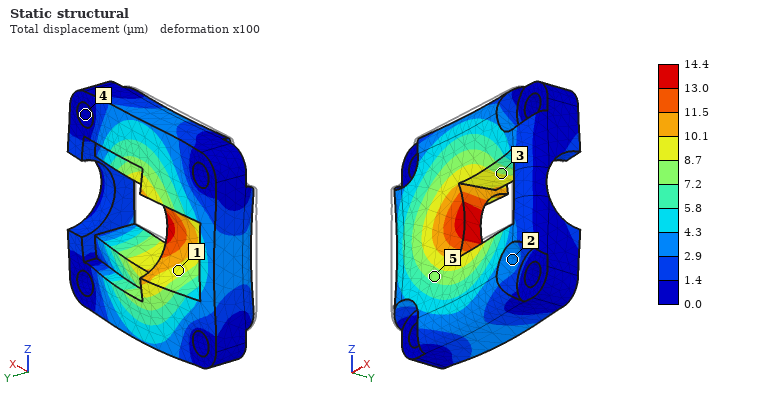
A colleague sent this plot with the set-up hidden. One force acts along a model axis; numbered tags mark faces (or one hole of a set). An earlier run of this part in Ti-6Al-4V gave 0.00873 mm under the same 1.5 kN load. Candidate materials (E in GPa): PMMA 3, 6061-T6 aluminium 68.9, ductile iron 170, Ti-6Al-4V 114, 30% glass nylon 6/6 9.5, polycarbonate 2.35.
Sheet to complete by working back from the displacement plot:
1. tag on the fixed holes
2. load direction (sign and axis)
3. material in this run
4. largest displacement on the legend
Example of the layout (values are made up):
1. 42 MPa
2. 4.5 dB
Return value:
1. 4
2. +Y
3. 6061-T6 aluminium
4. 14.4 µm
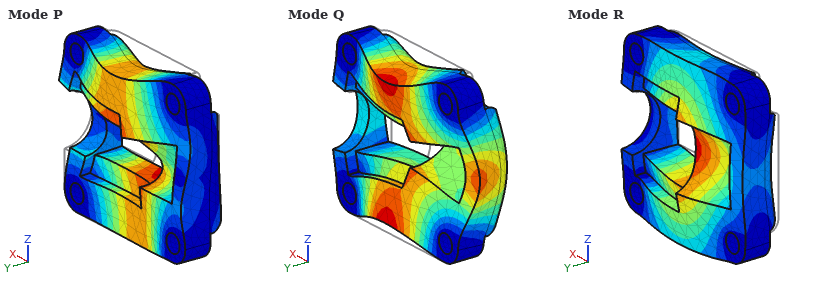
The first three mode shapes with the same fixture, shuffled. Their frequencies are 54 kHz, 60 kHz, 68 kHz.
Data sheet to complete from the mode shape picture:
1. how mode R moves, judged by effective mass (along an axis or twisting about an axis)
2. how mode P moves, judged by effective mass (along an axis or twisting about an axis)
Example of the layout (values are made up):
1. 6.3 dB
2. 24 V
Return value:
1. along Y
2. along Z
